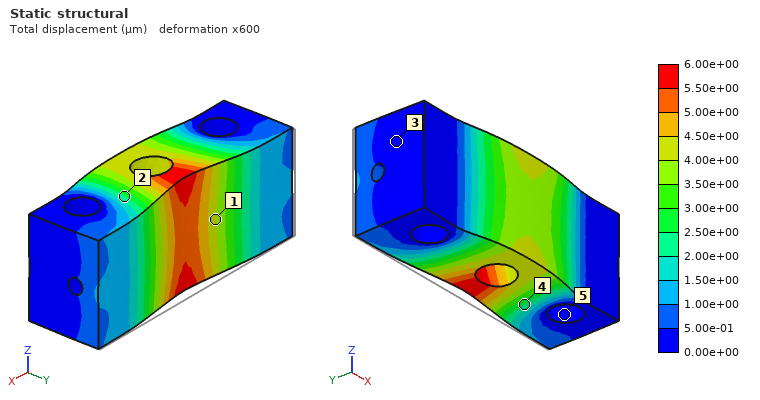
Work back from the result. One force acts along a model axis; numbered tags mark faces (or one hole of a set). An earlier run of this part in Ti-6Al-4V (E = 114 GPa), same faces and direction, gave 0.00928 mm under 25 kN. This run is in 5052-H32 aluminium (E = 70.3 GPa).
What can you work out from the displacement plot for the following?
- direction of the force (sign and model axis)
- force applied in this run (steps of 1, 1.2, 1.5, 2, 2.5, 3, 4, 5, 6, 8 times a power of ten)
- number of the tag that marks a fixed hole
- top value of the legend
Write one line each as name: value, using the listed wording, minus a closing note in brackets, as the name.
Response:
direction of the force: -Y
force applied in this run: 10 kN
number of the tag that marks a fixed hole: 5
top value of the legend: 6.00e+00 µm
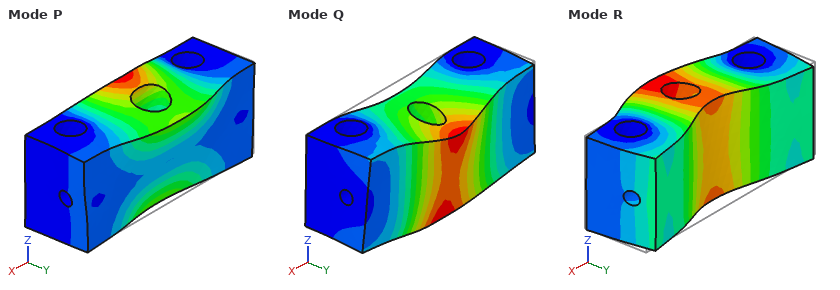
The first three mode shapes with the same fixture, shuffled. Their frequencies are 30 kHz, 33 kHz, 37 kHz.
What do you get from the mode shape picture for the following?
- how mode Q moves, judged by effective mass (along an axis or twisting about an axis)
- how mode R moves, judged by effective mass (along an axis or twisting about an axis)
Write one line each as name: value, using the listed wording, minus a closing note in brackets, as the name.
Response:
how mode Q moves, judged by effective mass: along Z
how mode R moves, judged by effective mass: along Y
